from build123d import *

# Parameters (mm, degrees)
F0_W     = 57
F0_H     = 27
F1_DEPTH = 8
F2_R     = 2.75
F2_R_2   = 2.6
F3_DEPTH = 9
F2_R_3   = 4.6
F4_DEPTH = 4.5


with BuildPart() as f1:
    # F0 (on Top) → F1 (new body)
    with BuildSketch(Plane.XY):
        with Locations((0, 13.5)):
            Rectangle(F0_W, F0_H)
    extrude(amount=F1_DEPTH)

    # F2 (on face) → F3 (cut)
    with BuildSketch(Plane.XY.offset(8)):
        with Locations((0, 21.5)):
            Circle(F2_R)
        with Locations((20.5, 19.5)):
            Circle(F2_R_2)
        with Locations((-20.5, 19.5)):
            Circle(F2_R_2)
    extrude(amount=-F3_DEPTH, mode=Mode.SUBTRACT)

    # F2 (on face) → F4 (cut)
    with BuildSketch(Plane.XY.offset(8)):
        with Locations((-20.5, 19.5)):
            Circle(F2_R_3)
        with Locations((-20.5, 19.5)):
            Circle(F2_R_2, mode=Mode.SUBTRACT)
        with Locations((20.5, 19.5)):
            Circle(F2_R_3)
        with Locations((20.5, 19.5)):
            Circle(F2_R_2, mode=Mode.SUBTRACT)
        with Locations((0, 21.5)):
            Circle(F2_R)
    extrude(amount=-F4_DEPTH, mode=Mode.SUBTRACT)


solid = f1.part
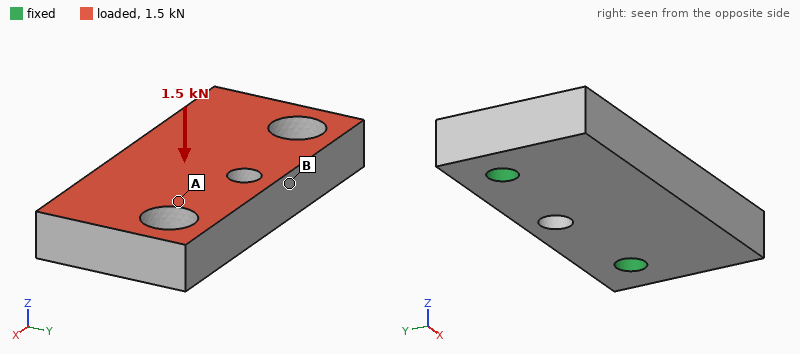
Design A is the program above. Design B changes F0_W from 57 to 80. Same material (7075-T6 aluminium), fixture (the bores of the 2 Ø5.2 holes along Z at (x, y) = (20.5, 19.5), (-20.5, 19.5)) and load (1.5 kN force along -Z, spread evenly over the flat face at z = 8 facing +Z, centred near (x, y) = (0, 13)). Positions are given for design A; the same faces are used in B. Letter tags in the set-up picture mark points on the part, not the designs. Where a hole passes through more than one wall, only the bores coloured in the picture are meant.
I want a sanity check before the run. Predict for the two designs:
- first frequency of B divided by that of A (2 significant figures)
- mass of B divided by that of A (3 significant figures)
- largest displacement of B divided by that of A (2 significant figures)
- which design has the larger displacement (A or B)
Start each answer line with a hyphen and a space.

- 0.90
- 1.44
- 0.86
- A
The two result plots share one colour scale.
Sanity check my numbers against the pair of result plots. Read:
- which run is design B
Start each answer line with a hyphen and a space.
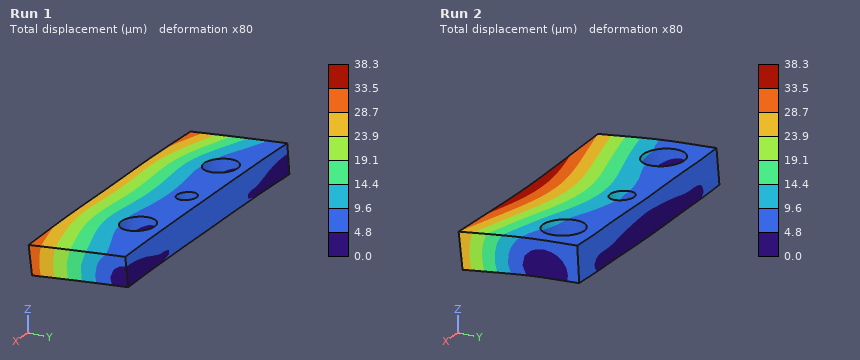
- Run 1
